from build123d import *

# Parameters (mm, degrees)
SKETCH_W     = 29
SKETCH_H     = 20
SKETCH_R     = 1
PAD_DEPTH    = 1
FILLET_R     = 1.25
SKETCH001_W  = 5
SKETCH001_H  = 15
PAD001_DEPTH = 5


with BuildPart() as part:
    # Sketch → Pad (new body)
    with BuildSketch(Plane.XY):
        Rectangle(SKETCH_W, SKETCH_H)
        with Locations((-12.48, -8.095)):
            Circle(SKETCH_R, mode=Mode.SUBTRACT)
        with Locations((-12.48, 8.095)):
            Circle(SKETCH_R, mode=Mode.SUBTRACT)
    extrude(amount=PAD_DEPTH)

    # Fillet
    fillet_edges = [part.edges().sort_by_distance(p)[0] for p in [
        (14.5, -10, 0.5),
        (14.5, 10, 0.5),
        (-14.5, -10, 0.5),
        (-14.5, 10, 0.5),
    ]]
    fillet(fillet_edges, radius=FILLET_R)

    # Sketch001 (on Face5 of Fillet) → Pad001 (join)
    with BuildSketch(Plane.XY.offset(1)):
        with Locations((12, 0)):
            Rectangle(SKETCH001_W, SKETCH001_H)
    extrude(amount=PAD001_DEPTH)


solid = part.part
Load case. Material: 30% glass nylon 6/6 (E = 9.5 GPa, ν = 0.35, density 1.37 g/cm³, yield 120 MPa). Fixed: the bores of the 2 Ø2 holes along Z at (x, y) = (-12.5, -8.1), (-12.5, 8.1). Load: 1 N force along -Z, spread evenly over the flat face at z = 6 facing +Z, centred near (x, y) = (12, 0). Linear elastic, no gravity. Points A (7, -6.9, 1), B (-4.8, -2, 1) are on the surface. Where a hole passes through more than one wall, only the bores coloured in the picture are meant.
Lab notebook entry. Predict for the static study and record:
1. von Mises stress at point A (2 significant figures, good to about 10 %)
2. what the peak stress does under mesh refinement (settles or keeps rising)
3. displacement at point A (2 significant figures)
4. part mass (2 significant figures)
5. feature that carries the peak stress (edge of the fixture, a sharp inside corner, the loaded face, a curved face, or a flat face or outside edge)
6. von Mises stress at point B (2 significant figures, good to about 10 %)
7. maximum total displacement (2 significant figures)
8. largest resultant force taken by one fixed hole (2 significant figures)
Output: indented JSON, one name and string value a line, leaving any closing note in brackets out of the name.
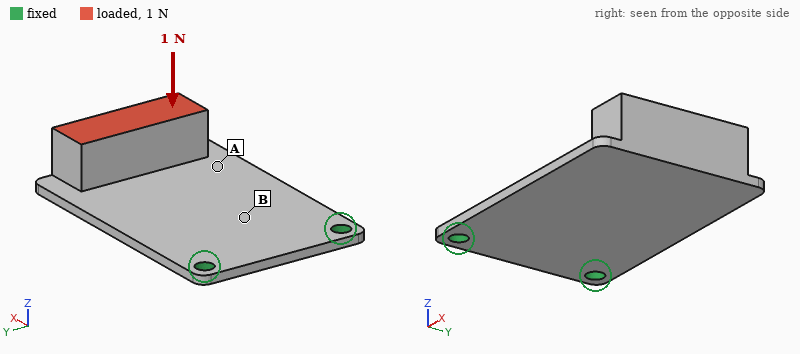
{
  "von Mises stress at point A": "1.6 MPa",
  "what the peak stress does under mesh refinement": "keeps rising",
  "displacement at point A": "0.23 mm",
  "part mass": "1.3 g",
  "feature that carries the peak stress": "edge of the fixture",
  "von Mises stress at point B": "4.6 MPa",
  "maximum total displacement": "0.39 mm",
  "largest resultant force taken by one fixed hole": "0.50 N"
}
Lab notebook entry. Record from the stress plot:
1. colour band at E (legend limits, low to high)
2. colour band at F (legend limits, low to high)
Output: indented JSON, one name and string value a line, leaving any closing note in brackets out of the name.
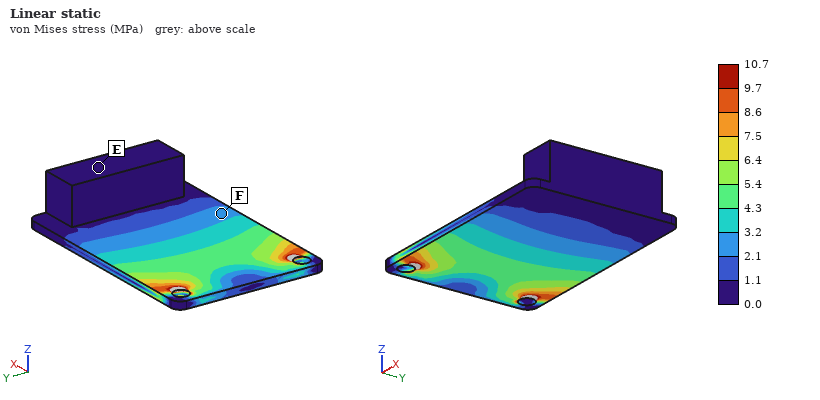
{
  "colour band at E": "0.0 to 1.1 MPa",
  "colour band at F": "2.1 to 3.2 MPa"
}
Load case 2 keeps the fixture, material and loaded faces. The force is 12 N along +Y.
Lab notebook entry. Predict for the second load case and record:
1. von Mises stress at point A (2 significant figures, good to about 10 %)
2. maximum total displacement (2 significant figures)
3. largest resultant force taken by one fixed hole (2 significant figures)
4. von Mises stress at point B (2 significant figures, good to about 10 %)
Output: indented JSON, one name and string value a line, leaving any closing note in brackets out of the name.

{
  "von Mises stress at point A": "13 MPa",
  "maximum total displacement": "0.37 mm",
  "largest resultant force taken by one fixed hole": "19 N",
  "von Mises stress at point B": "14 MPa"
}
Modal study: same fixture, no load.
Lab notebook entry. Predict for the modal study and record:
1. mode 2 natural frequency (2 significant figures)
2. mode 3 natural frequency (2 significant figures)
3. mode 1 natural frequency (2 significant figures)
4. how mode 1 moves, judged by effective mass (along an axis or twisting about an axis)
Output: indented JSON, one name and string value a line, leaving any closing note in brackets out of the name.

{
  "mode 2 natural frequency": "1300 Hz",
  "mode 3 natural frequency": "2500 Hz",
  "mode 1 natural frequency": "320 Hz",
  "how mode 1 moves, judged by effective mass": "along Z"
}
